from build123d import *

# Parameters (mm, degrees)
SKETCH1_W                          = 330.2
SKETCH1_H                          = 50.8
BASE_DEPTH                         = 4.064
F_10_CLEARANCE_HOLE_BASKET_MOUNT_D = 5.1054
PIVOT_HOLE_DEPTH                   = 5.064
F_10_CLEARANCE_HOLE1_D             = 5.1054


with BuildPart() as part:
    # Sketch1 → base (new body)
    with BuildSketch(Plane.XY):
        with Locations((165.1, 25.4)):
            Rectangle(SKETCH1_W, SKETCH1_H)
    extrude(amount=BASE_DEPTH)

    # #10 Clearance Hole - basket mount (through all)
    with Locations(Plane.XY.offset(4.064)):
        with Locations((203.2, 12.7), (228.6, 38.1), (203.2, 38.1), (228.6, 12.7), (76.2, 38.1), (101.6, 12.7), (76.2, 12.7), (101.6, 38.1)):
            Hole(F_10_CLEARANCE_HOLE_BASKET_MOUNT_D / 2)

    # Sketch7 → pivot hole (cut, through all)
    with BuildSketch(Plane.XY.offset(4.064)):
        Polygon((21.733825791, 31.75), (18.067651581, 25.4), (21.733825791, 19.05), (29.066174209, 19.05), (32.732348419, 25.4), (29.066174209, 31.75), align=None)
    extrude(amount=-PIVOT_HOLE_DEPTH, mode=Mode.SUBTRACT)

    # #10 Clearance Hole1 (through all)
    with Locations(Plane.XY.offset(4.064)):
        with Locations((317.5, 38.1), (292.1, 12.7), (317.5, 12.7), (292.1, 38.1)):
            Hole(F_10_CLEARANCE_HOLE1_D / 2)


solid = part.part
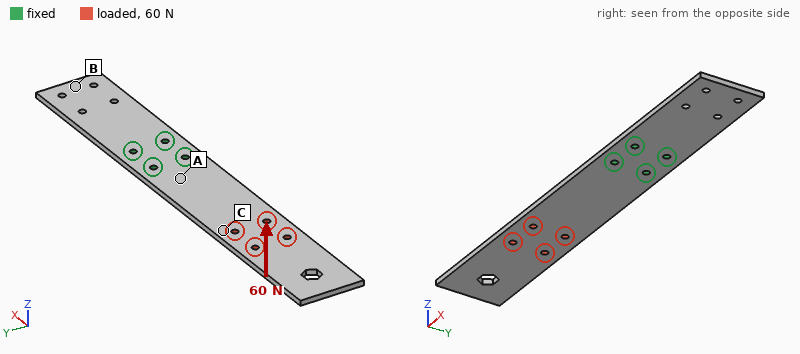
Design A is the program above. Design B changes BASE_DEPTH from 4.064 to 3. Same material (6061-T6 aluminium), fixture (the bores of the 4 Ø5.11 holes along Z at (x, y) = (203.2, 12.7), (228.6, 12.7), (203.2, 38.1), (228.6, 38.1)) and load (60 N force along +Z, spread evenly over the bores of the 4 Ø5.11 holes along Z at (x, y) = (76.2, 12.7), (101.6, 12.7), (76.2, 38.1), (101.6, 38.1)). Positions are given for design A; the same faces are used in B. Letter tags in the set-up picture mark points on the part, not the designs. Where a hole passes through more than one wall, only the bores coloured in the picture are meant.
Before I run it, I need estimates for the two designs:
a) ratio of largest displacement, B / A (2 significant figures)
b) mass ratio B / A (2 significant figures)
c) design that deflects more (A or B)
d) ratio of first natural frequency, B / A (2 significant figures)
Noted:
2.5
0.74
B
0.74
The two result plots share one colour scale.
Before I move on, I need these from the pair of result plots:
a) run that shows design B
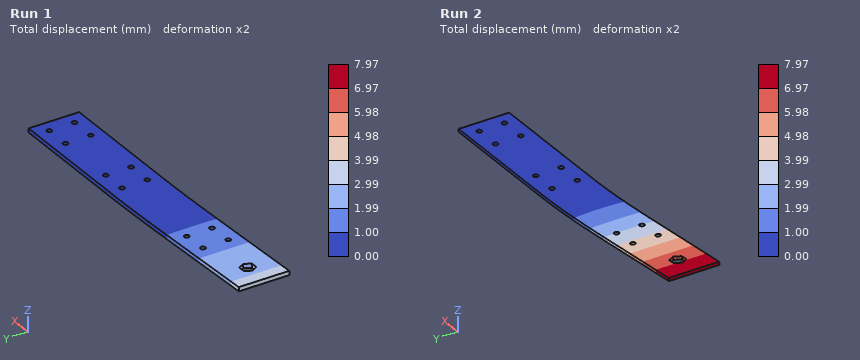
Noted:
Run 2
